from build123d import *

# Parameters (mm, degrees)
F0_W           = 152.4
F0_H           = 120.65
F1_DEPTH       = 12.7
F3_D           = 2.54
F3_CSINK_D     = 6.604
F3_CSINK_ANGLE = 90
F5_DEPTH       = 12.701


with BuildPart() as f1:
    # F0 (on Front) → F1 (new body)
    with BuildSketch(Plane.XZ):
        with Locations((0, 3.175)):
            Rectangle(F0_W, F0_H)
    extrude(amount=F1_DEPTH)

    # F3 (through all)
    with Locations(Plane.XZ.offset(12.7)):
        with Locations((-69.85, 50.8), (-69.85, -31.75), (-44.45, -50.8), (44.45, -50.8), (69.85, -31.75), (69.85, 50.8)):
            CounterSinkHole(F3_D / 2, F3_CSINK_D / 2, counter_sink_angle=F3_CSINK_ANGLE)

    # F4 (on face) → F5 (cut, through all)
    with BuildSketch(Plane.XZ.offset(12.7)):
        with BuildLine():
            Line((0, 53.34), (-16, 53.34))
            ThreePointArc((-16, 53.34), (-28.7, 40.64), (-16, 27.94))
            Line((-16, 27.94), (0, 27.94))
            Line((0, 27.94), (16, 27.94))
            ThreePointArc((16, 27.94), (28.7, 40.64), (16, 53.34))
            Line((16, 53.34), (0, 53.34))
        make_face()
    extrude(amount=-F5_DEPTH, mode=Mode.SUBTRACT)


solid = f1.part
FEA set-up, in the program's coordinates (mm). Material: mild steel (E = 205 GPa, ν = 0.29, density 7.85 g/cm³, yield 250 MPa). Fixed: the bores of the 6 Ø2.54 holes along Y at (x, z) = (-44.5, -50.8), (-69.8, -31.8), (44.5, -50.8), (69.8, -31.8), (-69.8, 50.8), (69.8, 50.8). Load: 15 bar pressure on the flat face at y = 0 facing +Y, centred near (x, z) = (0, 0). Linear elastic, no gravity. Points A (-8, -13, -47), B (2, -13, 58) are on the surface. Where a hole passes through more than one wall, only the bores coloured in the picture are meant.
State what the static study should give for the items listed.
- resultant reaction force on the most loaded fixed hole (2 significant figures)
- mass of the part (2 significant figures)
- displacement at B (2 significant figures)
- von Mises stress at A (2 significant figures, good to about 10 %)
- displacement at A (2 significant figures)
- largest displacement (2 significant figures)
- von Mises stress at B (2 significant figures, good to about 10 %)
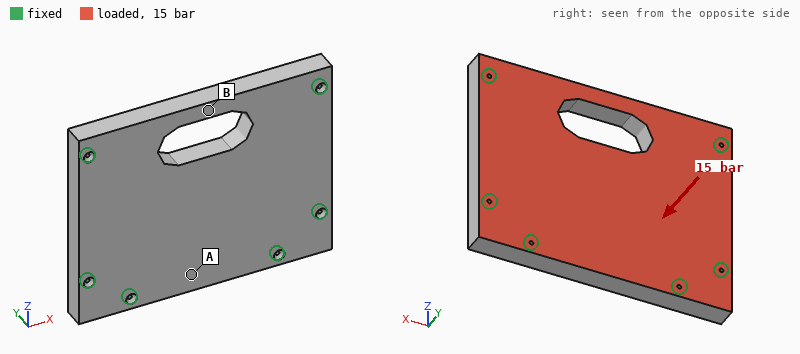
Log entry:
5.5 kN
1.7 kg
84 µm
39 MPa
27 µm
89 µm
76 MPa
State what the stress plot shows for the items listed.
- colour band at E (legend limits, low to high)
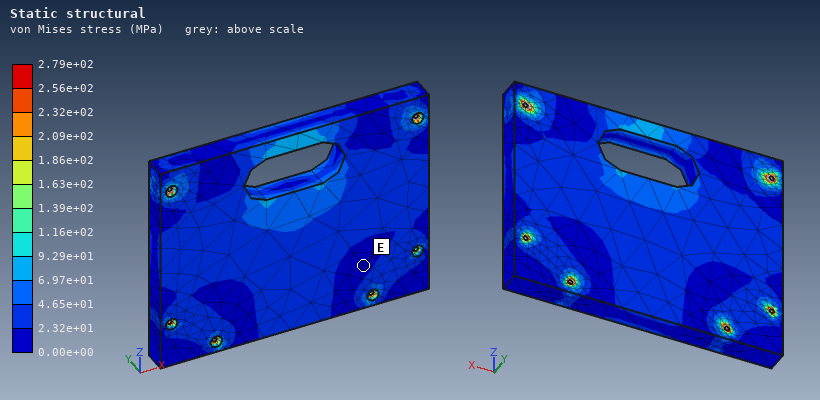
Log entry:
0.00e+00 to 2.32e+01 MPa
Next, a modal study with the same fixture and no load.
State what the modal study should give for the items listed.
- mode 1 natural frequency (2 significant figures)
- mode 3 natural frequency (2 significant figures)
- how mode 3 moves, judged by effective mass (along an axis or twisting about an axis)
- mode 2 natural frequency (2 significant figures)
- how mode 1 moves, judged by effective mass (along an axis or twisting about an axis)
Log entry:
2600 Hz
5800 Hz
twisting about Z
4700 Hz
along Y
